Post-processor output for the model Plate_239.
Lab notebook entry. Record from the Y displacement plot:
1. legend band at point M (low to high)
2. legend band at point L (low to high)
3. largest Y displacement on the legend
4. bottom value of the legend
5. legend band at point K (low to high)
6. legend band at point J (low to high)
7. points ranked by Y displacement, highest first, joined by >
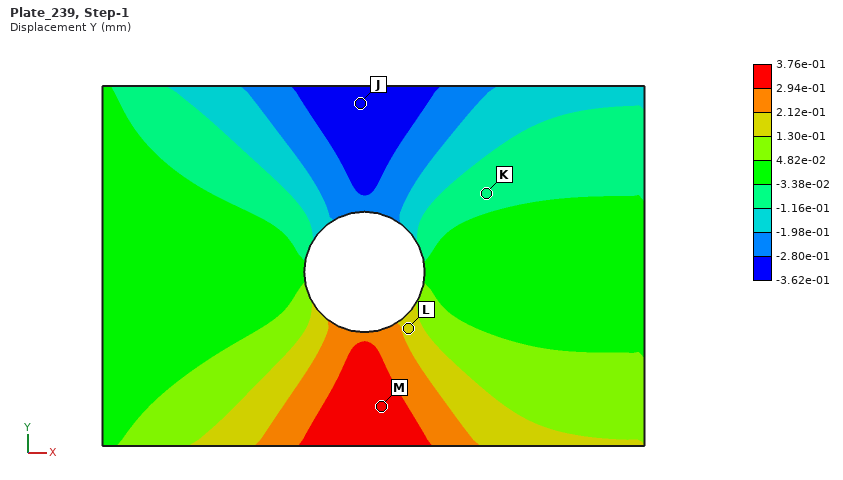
2.94e-01 to 3.76e-01 mm
1.30e-01 to 2.12e-01 mm
3.76e-01 mm
-3.62e-01 mm
-1.16e-01 to -3.38e-02 mm
-3.62e-01 to -2.80e-01 mm
M > L > K > J
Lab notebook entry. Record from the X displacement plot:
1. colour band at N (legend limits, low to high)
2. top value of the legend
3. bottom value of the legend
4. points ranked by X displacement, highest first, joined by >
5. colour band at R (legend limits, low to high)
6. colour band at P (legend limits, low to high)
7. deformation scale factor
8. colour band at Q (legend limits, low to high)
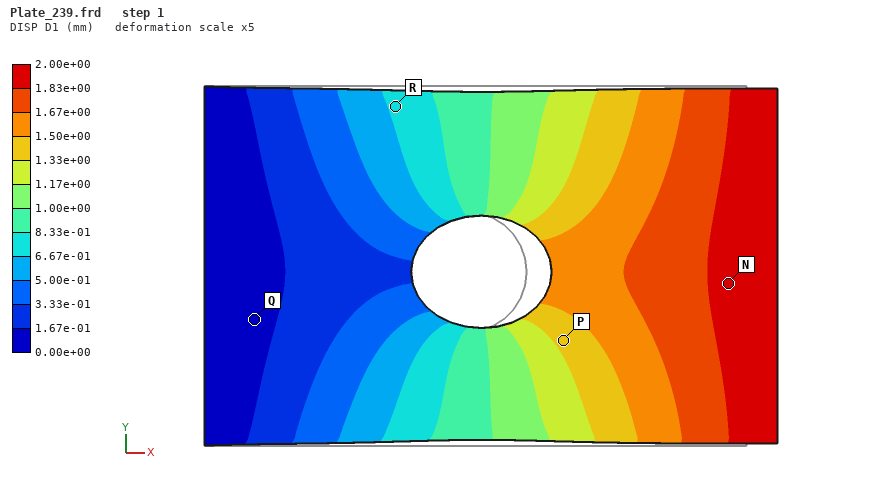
1.83e+00 to 2.00e+00 mm
2.00e+00 mm
0.00e+00 mm
N > P > R > Q
6.67e-01 to 8.33e-01 mm
1.33e+00 to 1.50e+00 mm
5
0.00e+00 to 1.67e-01 mm
